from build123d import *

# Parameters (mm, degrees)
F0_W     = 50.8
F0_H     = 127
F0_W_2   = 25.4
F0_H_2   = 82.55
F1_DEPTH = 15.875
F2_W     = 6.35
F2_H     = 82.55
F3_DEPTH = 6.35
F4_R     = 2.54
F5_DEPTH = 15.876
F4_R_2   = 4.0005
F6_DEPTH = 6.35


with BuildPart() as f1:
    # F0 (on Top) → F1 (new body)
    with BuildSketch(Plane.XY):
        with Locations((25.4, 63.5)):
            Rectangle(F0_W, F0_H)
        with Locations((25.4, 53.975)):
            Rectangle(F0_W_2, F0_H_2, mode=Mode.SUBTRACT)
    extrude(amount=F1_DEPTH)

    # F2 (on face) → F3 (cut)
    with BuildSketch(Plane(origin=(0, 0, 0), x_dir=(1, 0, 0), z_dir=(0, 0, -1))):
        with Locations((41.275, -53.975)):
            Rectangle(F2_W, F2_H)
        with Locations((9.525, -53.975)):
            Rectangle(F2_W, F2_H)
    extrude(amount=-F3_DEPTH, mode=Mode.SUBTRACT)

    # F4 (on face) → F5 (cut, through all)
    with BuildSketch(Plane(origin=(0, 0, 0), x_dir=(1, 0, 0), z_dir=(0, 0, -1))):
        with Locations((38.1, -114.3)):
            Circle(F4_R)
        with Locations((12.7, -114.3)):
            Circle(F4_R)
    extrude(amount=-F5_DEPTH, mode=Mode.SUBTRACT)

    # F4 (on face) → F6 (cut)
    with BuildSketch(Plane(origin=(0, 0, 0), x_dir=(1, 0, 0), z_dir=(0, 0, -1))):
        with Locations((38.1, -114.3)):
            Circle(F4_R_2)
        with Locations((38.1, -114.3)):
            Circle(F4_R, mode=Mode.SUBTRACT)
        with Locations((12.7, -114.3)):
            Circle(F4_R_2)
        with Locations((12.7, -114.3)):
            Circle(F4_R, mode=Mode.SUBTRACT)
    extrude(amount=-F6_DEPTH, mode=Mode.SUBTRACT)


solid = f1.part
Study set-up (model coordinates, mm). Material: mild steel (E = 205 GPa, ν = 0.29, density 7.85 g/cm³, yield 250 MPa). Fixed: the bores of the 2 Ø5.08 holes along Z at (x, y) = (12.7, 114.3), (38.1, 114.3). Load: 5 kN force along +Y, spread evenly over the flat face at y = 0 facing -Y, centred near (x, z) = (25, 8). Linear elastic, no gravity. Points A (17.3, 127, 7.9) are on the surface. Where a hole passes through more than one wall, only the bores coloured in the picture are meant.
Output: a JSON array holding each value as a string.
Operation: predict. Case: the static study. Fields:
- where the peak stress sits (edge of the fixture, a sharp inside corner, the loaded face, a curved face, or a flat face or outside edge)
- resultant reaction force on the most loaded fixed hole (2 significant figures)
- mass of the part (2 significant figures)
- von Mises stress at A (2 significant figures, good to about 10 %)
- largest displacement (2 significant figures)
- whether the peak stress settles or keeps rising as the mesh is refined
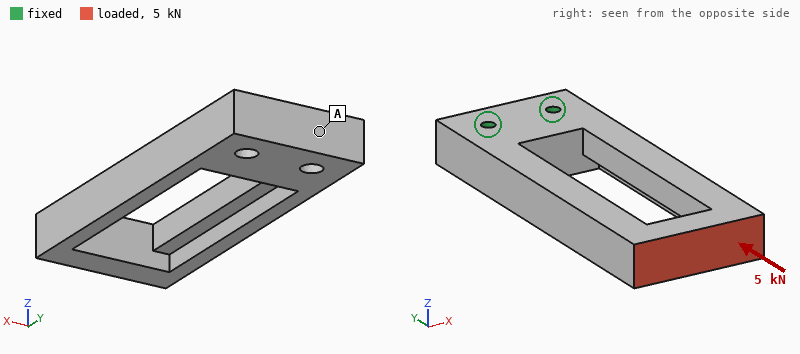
["edge of the fixture", "2.5 kN", "480 g", "6.1 MPa", "44 µm", "keeps rising"]
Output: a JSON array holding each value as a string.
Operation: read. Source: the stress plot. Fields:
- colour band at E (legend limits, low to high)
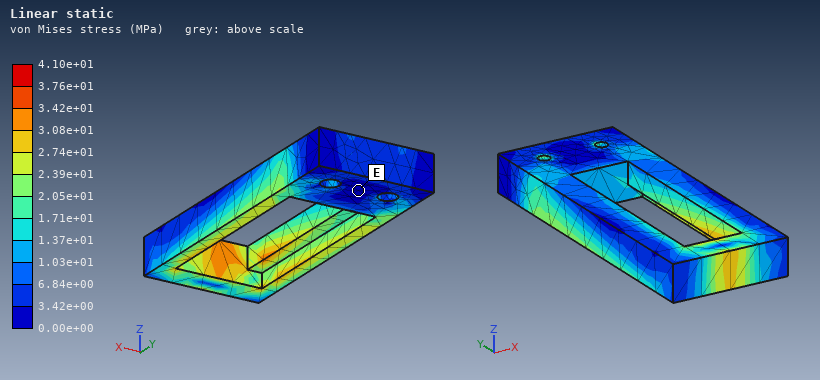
["0.00e+00 to 3.42e+00 MPa"]
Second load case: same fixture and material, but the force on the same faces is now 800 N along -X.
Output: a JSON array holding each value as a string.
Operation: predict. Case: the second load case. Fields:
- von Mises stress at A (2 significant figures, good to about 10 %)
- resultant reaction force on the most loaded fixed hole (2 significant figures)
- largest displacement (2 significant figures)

["7.7 MPa", "3.2 kN", "0.10 mm"]
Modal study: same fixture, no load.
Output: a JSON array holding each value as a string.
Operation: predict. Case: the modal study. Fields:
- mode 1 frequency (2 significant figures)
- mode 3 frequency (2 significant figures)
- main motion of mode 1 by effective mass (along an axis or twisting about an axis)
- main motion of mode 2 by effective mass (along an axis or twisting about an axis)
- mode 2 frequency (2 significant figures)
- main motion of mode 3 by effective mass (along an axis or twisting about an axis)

["750 Hz", "2100 Hz", "along Z", "along X", "1200 Hz", "twisting about Y"]
